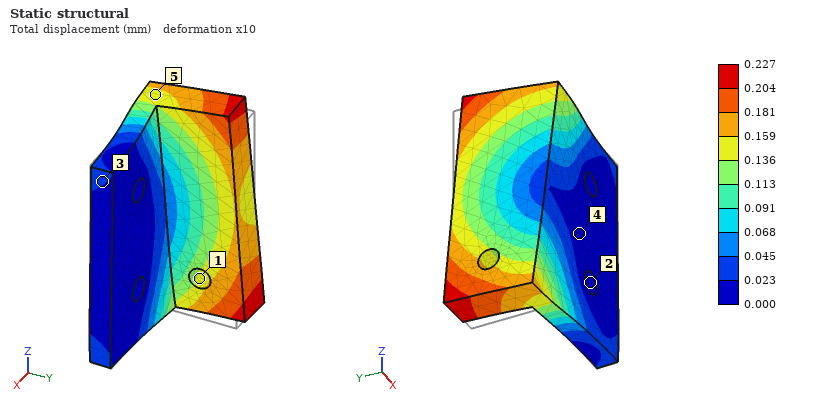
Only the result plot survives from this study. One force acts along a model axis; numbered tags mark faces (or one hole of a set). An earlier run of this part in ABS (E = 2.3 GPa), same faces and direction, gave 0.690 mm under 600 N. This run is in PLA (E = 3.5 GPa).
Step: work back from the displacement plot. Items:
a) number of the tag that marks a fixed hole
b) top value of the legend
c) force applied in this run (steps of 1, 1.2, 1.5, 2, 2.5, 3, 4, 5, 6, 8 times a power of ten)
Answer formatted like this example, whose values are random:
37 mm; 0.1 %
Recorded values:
2; 0.227 mm; 300 N
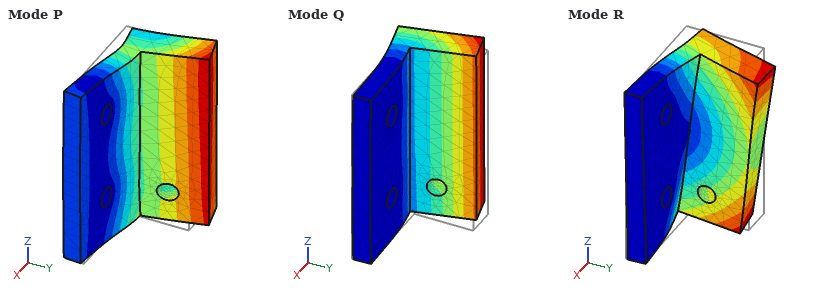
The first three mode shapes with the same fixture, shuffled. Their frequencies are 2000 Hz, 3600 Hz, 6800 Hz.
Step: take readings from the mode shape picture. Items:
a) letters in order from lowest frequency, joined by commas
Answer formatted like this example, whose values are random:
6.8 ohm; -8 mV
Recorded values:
Q, R, P
